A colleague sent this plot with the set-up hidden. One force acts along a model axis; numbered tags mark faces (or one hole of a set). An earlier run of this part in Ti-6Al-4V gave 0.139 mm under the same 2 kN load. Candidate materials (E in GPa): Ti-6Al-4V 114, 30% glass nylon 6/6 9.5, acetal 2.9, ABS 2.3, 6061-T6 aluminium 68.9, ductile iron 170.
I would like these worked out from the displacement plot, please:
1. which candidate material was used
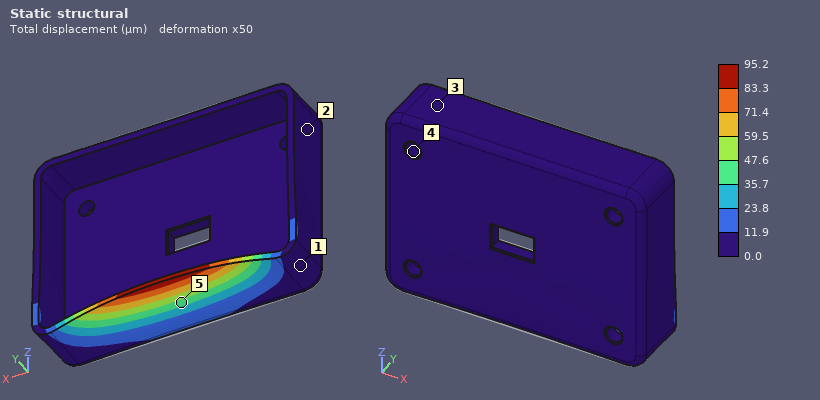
ductile iron
